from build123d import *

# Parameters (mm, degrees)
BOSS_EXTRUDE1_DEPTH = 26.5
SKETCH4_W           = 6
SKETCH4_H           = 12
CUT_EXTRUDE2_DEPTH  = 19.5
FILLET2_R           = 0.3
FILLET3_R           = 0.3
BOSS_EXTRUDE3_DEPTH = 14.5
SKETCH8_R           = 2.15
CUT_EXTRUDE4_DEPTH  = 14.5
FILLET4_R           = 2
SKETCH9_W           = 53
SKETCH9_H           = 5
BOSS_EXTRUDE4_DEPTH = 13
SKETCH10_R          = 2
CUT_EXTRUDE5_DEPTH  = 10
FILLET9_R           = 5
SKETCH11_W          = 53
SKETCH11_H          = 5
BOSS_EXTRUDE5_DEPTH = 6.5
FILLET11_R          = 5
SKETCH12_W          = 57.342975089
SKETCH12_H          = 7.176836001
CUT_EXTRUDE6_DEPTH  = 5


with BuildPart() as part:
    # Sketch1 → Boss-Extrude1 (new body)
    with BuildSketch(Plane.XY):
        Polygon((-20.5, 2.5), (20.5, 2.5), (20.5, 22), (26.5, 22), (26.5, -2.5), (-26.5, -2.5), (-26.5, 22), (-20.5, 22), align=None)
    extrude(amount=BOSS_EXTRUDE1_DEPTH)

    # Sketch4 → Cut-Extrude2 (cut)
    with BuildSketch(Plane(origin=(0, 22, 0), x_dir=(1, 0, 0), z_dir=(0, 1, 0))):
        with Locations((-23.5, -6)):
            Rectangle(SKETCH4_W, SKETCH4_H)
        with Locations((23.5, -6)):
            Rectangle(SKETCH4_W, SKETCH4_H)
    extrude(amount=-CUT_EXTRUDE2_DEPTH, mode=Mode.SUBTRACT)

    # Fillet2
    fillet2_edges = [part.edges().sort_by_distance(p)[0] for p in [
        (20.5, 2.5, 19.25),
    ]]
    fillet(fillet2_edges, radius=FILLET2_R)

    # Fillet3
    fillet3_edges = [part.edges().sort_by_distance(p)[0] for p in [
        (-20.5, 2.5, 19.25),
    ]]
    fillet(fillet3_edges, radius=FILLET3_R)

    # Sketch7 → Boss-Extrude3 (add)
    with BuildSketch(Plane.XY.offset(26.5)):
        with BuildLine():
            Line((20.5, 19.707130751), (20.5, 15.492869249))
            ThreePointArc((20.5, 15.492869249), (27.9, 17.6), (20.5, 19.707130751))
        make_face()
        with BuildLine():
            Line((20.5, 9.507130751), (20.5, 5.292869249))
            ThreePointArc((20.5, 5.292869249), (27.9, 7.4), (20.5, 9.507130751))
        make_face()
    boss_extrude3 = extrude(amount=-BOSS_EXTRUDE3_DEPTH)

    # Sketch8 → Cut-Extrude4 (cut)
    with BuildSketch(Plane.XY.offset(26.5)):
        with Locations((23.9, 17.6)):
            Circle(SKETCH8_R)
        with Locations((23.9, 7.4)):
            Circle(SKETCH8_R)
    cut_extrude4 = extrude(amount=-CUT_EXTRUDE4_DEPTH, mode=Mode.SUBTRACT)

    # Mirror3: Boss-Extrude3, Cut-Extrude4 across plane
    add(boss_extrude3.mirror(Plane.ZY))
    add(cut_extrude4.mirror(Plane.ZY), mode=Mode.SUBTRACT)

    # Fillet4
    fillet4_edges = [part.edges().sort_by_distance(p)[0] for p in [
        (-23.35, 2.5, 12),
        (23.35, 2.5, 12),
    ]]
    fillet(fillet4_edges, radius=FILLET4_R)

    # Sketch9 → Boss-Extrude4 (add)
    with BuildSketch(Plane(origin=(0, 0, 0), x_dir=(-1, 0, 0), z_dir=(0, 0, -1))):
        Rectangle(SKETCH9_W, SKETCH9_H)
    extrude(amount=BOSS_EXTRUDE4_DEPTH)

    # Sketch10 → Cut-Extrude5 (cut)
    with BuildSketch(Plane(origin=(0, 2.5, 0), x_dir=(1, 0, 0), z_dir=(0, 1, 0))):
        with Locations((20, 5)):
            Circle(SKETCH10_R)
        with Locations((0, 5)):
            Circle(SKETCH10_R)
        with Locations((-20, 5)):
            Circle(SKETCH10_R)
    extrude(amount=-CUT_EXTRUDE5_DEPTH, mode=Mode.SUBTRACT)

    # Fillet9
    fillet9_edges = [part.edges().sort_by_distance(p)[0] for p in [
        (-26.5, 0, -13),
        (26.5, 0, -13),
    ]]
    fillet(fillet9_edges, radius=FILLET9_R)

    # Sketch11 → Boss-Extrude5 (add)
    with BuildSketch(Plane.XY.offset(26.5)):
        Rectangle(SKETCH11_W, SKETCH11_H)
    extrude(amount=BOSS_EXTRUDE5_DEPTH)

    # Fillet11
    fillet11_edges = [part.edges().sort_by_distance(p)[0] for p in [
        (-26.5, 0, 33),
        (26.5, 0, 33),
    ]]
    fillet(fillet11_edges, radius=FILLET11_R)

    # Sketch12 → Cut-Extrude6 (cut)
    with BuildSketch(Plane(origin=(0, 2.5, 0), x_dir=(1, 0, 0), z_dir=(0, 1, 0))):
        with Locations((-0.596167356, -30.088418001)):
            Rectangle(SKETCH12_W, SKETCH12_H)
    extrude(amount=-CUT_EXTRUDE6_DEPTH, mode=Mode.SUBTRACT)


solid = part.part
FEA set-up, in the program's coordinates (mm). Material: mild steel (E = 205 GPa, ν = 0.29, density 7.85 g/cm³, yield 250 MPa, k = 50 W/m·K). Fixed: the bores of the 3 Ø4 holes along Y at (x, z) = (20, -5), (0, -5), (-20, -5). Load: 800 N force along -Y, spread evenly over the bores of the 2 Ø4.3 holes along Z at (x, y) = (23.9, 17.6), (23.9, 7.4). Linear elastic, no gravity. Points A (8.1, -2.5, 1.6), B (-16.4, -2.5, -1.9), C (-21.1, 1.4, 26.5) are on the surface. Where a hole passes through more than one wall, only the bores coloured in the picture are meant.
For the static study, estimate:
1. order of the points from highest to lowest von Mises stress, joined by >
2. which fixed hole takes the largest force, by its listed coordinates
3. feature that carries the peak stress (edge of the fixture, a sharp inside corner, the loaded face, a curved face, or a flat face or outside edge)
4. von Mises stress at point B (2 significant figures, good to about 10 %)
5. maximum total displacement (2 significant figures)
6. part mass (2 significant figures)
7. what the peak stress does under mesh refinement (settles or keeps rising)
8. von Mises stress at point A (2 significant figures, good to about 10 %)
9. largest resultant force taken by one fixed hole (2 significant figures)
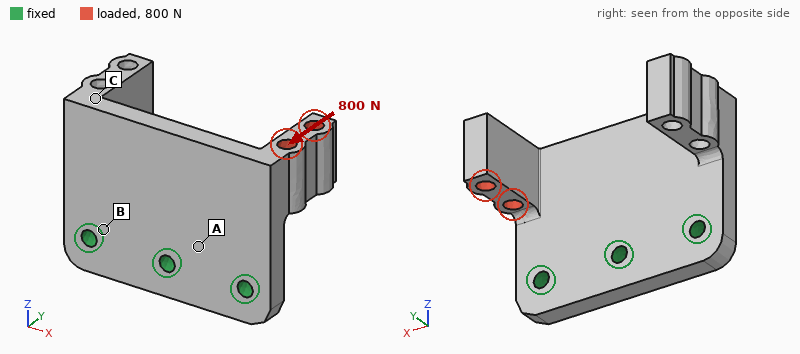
A > B > C
(20, -5)
edge of the fixture
30 MPa
0.13 mm
100 g
keeps rising
67 MPa
780 N
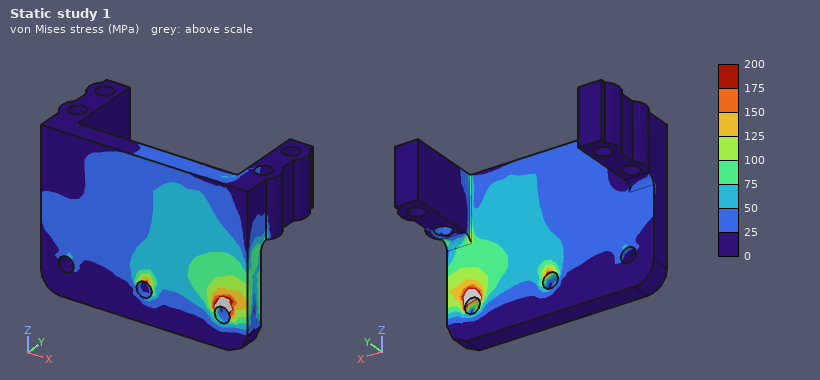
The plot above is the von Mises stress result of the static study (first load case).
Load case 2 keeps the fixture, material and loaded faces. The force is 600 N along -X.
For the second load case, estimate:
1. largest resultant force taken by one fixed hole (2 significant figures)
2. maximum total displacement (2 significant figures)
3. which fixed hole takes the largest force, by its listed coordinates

490 N
69 µm
(20, -5)
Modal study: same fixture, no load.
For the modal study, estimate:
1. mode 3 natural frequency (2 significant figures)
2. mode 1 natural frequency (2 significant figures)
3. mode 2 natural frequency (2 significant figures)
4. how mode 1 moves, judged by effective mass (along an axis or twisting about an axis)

5300 Hz
2800 Hz
3600 Hz
along Y
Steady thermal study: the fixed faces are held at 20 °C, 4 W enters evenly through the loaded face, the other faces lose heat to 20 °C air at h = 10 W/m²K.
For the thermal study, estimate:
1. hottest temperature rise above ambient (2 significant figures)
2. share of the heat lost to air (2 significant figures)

27 K
9.7 %
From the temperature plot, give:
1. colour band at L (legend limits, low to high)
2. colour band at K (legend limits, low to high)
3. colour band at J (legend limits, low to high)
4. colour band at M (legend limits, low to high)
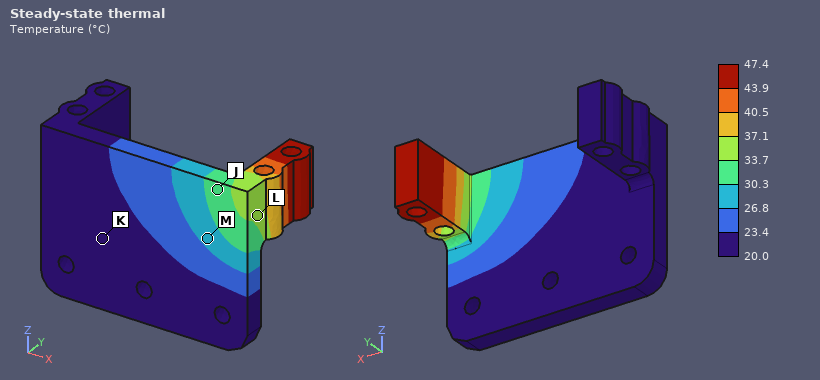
33.7 to 37.1 °C
20.0 to 23.4 °C
30.3 to 33.7 °C
26.8 to 30.3 °C
